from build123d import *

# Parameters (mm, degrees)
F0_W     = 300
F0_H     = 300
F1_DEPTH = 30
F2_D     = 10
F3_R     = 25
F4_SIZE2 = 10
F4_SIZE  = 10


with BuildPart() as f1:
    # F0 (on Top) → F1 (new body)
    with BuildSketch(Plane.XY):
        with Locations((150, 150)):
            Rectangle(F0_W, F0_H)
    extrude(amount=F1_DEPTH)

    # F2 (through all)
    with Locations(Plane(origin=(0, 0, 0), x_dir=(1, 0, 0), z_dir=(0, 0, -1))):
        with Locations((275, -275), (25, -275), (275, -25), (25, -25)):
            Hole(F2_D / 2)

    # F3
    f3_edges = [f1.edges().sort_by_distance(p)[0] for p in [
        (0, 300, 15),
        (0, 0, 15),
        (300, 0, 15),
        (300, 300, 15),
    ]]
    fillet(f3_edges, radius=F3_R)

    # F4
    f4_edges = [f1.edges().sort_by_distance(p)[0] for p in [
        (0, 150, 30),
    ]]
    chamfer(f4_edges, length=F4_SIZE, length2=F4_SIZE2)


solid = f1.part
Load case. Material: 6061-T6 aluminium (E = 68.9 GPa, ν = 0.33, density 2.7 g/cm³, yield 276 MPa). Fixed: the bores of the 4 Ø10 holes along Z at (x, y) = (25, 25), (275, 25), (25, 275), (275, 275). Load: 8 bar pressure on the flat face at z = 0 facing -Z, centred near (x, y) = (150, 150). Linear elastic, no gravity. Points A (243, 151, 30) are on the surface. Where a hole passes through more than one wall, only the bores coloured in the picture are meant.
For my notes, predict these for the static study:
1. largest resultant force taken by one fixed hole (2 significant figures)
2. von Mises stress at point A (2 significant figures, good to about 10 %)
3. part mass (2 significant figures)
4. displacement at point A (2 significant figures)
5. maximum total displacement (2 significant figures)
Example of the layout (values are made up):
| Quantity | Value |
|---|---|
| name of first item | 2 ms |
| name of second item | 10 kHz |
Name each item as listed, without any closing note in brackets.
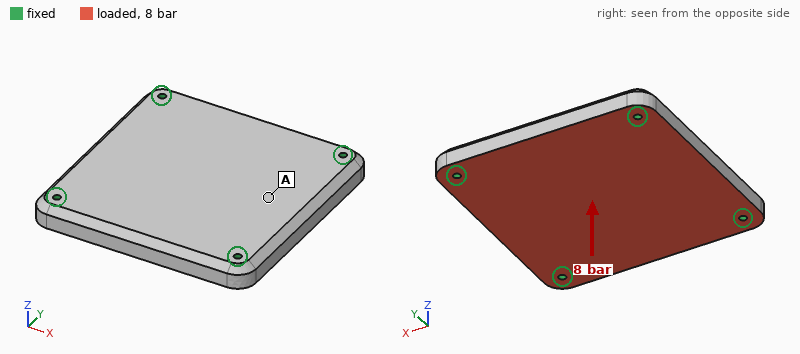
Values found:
| Quantity | Value |
|---|---|
| largest resultant force taken by one fixed hole | 18 kN |
| von Mises stress at point A | 20 MPa |
| part mass | 7.1 kg |
| displacement at point A | 0.15 mm |
| maximum total displacement | 0.20 mm |
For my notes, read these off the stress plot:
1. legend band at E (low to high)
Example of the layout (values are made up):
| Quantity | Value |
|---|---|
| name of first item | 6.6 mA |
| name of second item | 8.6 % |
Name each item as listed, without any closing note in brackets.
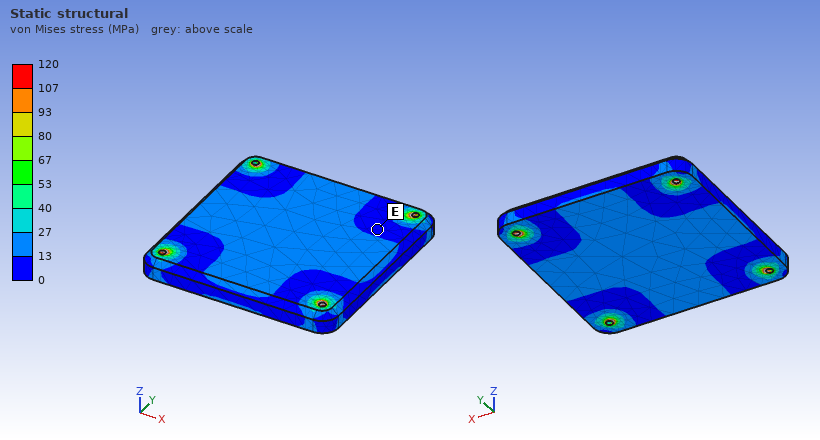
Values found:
| Quantity | Value |
|---|---|
| legend band at E | 0 to 13 MPa |
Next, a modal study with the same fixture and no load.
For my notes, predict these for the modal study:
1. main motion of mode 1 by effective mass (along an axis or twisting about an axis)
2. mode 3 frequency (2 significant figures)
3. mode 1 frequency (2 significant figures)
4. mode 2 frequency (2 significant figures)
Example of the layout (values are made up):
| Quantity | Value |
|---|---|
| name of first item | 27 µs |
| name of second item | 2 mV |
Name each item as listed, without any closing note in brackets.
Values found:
| Quantity | Value |
|---|---|
| main motion of mode 1 by effective mass | along Z |
| mode 3 frequency | 2300 Hz |
| mode 1 frequency | 1400 Hz |
| mode 2 frequency | 2300 Hz |
